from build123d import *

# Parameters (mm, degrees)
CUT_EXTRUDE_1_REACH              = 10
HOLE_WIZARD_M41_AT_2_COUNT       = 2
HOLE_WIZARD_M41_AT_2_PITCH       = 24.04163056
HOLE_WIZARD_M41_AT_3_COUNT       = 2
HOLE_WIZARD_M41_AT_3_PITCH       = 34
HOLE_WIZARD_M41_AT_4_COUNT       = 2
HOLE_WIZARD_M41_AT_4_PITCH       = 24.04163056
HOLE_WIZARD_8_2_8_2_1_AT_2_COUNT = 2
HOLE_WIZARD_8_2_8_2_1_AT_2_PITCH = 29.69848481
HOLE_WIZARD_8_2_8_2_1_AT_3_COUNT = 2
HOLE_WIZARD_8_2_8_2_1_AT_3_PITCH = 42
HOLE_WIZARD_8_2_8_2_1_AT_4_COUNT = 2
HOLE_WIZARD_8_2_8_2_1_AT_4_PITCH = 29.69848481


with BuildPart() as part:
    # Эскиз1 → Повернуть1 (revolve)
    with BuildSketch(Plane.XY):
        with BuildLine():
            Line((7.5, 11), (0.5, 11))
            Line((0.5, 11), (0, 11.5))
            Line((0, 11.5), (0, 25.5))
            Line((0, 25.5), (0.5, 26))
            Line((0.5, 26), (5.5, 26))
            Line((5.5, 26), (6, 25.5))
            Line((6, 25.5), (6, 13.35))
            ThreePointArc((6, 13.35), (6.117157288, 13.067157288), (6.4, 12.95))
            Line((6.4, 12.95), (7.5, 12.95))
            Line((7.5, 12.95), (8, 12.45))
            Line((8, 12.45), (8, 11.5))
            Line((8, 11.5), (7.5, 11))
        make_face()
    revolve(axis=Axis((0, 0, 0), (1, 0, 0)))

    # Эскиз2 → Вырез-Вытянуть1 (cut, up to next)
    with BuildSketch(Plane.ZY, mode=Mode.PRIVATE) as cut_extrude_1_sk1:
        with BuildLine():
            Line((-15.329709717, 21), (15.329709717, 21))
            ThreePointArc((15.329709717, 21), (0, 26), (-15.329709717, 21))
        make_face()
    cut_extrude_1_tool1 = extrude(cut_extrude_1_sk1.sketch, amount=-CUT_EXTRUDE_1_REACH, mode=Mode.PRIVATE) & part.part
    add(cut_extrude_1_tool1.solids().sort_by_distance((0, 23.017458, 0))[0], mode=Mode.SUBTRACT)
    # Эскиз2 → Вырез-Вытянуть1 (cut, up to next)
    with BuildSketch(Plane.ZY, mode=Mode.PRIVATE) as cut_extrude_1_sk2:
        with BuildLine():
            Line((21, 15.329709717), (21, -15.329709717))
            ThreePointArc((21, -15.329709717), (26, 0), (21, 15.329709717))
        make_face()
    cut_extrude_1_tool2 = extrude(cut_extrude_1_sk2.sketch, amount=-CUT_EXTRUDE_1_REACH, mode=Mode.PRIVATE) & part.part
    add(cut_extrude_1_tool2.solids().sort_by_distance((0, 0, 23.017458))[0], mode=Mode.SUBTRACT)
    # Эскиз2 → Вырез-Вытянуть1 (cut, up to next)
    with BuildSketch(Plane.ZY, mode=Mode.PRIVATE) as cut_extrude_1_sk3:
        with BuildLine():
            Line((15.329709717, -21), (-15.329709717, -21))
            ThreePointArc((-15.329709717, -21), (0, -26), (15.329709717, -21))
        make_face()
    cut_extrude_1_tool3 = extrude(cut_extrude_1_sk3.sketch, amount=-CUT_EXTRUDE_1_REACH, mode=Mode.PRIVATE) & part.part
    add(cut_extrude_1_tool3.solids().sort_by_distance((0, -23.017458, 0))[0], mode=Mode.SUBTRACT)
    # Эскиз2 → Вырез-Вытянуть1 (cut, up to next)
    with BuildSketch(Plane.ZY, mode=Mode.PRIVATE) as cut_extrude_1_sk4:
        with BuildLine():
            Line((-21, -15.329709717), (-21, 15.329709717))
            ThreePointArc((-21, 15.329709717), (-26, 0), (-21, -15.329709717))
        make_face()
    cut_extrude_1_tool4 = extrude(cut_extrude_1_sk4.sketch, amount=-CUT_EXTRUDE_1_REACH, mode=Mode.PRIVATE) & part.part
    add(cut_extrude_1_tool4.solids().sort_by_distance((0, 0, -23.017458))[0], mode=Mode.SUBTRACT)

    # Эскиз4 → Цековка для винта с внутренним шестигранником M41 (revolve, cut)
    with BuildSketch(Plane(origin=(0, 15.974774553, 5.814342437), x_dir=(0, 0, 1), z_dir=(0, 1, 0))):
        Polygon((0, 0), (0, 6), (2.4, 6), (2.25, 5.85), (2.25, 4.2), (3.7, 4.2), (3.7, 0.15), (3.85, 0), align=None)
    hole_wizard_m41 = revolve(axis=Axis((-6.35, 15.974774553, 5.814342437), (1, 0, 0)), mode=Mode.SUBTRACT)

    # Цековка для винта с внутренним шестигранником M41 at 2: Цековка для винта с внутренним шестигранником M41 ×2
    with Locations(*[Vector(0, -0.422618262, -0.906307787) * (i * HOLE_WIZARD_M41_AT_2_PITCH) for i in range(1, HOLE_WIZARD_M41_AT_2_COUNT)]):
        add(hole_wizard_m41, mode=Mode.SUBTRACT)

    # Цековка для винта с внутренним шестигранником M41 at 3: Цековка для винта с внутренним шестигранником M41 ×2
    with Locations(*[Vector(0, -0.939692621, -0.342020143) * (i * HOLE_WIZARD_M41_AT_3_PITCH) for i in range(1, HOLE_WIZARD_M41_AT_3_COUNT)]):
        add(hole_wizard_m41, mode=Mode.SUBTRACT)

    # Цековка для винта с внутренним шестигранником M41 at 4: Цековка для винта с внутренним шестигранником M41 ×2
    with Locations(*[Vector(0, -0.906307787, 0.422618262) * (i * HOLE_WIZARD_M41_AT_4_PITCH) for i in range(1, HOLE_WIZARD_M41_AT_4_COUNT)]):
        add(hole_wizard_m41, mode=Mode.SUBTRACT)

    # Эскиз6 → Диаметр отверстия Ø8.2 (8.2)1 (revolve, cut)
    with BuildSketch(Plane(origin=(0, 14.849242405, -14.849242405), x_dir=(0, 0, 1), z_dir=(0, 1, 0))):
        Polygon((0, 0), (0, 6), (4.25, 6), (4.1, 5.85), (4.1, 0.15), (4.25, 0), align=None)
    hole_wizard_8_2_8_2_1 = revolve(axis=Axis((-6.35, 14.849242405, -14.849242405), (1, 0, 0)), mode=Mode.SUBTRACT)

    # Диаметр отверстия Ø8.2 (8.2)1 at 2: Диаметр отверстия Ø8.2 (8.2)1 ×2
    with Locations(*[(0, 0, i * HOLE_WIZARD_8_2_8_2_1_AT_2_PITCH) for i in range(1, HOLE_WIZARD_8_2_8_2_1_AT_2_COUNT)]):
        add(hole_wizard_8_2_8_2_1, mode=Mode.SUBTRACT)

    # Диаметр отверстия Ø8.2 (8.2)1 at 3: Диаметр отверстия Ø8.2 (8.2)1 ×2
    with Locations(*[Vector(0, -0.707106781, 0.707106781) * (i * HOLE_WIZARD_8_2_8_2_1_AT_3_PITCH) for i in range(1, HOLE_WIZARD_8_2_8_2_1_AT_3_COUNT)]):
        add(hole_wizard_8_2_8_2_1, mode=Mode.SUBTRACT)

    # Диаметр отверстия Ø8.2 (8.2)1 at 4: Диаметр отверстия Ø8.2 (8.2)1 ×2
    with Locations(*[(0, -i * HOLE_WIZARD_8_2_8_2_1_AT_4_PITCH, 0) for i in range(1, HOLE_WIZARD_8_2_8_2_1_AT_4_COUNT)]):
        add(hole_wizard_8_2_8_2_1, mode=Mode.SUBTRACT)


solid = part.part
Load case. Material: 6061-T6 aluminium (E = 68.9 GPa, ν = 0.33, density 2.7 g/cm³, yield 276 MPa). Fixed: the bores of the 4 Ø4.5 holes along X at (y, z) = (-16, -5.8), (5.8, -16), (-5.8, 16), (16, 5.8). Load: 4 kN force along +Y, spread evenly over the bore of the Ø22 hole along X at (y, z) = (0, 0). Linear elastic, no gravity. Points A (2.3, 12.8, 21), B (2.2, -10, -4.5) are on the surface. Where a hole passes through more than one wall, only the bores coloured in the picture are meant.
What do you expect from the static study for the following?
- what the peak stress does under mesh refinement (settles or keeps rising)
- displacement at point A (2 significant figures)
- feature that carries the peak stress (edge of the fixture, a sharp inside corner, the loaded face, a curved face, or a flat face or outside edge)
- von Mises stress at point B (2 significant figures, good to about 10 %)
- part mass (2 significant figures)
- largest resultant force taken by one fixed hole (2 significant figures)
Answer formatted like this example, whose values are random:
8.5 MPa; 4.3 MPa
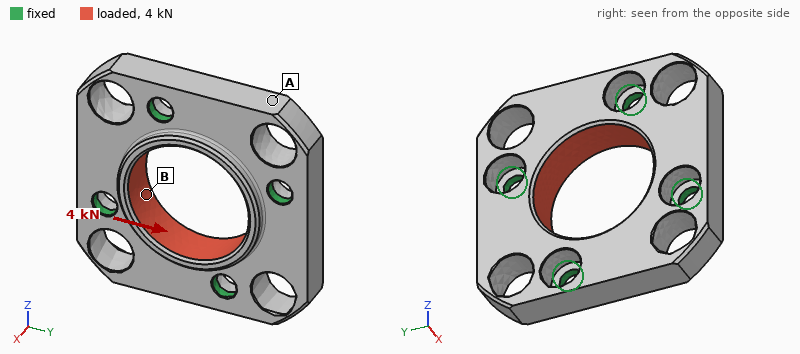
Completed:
keeps rising; 4.3 µm; edge of the fixture; 27 MPa; 16 g; 1.0 kN
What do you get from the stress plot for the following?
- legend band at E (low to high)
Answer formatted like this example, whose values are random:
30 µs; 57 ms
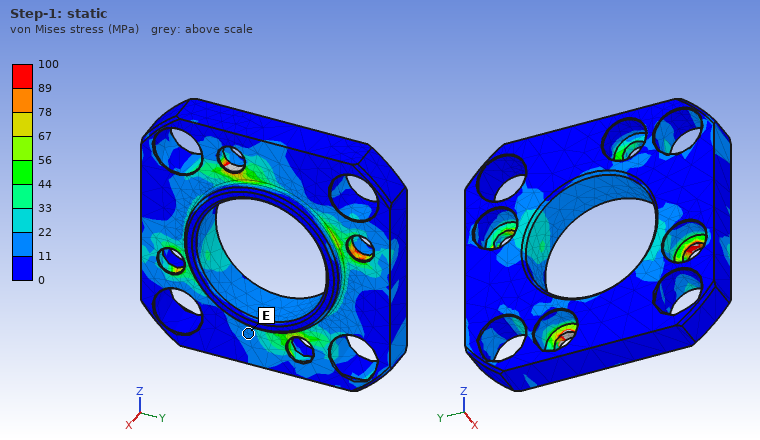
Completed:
11 to 22 MPa
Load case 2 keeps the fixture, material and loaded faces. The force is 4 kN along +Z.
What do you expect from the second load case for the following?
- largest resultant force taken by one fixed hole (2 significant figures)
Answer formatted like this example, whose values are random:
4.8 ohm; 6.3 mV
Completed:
1.0 kN
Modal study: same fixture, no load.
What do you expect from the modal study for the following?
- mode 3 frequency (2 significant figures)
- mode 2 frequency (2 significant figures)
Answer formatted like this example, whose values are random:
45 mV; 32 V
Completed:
18 kHz; 18 kHz
